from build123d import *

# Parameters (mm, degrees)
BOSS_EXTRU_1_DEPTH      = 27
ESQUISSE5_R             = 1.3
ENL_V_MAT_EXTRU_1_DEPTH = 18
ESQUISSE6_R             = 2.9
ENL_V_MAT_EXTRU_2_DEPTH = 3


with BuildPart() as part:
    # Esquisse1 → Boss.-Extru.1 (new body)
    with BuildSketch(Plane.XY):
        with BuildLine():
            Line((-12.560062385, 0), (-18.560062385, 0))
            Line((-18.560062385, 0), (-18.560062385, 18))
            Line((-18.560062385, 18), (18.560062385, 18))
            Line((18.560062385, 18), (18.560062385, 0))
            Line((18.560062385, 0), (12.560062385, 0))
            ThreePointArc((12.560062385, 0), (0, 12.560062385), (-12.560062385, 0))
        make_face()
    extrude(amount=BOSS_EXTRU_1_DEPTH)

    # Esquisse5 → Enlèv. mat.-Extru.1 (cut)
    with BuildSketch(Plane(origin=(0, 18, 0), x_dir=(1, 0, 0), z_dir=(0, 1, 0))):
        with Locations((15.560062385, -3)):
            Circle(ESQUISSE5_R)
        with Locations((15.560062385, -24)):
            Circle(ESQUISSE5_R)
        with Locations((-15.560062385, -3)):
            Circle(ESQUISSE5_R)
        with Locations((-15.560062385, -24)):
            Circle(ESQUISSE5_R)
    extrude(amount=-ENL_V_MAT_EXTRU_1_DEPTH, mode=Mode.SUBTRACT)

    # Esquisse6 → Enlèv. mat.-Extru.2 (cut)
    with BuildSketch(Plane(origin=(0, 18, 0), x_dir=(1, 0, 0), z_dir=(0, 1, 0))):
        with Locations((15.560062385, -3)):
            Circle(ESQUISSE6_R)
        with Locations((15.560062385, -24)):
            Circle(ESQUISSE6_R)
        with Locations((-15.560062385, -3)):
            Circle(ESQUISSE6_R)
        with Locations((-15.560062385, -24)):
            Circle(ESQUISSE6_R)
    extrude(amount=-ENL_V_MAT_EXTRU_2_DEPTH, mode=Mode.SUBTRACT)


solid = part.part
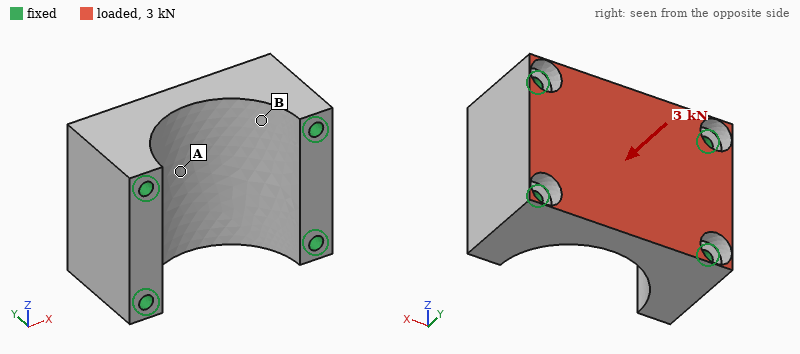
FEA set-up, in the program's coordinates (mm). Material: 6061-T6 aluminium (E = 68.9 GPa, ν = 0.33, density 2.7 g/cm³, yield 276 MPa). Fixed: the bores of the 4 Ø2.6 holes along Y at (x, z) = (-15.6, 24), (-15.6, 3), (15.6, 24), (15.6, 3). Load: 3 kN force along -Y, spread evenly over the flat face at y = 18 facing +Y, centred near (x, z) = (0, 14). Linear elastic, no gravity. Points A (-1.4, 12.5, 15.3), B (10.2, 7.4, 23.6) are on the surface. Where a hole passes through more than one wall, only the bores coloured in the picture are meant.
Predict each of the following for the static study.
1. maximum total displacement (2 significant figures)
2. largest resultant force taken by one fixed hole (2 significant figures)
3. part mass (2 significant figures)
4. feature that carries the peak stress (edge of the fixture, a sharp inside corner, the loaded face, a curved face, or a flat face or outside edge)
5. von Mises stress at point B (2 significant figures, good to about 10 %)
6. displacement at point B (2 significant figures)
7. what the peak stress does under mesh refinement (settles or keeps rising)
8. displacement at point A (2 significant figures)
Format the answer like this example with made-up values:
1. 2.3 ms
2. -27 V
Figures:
1. 4.3 µm
2. 870 N
3. 29 g
4. edge of the fixture
5. 17 MPa
6. 1.2 µm
7. keeps rising
8. 4.2 µm
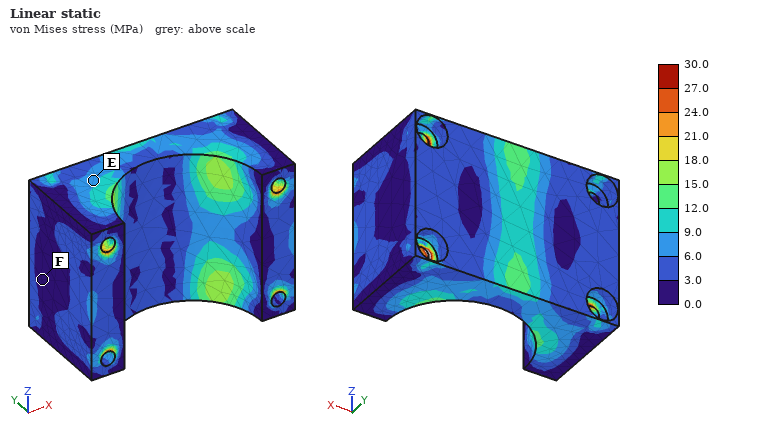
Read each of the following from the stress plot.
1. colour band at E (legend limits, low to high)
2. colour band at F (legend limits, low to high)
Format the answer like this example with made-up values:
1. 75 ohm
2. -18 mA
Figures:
1. 6.0 to 9.0 MPa
2. 0.0 to 3.0 MPa
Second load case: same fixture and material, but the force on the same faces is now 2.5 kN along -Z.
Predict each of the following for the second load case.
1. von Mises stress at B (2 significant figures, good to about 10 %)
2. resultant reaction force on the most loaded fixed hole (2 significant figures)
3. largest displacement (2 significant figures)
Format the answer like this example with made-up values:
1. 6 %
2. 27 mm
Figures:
1. 7.7 MPa
2. 830 N
3. 4.6 µm
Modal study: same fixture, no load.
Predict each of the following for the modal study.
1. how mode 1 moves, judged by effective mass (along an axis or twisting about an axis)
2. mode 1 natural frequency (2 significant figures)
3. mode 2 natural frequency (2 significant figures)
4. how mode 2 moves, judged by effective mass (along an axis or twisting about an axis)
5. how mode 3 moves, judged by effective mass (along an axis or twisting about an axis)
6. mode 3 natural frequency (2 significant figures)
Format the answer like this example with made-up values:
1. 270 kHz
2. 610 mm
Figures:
1. along Y
2. 37 kHz
3. 44 kHz
4. along Z
5. along X
6. 47 kHz
